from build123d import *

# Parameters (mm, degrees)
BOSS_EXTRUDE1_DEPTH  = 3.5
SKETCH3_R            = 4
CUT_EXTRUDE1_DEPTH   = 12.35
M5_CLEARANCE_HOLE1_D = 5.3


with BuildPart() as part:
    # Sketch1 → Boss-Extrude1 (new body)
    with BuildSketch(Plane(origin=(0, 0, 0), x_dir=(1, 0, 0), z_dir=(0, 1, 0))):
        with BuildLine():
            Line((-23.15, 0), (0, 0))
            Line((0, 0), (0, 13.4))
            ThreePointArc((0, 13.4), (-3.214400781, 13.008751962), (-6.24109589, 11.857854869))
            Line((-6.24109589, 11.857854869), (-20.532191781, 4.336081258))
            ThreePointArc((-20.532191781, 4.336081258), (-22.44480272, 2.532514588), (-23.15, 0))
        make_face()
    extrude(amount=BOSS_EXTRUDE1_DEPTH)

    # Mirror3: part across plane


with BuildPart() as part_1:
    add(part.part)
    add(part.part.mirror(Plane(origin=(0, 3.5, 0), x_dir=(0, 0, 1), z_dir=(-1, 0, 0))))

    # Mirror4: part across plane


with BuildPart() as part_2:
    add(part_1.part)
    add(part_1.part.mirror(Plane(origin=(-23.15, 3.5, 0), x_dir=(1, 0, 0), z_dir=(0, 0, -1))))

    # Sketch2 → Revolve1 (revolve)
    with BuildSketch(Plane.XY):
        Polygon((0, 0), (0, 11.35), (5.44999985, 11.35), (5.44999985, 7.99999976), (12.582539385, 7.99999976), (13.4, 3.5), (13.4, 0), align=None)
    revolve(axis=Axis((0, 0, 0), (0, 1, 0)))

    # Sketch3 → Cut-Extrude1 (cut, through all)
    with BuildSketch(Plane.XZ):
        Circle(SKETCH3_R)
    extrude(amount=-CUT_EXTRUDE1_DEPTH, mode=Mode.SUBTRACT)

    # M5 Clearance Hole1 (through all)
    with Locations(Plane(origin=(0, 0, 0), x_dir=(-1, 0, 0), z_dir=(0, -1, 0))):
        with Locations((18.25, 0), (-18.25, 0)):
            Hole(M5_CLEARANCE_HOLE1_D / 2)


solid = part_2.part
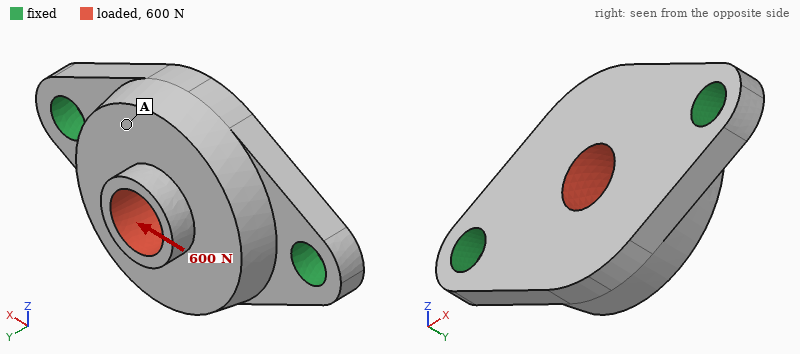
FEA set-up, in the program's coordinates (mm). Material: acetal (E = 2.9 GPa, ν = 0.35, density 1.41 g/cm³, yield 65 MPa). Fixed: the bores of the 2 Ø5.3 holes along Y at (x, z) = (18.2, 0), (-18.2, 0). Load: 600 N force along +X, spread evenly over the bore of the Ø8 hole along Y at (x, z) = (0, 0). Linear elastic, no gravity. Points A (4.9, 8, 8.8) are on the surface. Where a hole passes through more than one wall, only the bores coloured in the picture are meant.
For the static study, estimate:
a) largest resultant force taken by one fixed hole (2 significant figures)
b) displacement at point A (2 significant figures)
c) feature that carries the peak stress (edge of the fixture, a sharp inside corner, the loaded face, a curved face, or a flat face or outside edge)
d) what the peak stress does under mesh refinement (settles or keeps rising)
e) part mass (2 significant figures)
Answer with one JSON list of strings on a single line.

["310 N", "25 µm", "edge of the fixture", "keeps rising", "6.8 g"]
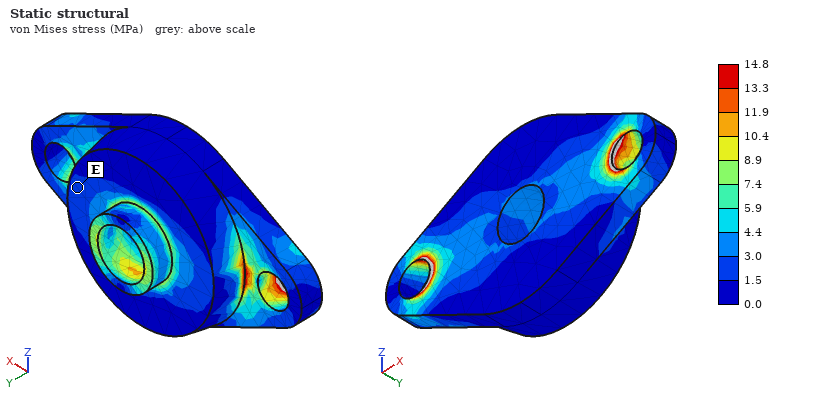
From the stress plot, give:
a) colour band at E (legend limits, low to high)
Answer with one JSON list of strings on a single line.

["1.5 to 3.0 MPa"]
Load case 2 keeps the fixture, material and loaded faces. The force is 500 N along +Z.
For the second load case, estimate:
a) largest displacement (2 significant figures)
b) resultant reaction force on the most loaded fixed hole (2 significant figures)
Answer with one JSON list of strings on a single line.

["0.30 mm", "250 N"]
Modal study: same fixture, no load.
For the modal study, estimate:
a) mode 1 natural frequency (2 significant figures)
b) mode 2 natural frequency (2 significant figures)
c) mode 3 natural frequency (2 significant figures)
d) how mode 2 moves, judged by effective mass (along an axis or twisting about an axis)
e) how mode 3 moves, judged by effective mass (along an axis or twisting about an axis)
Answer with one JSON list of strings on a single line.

["2700 Hz", "4300 Hz", "7500 Hz", "along Y", "along Z"]
